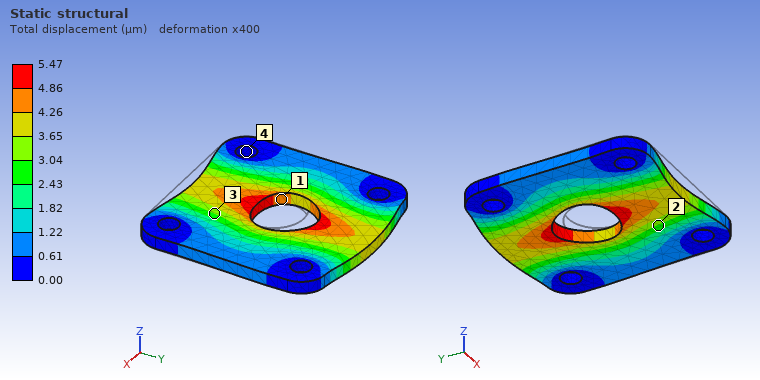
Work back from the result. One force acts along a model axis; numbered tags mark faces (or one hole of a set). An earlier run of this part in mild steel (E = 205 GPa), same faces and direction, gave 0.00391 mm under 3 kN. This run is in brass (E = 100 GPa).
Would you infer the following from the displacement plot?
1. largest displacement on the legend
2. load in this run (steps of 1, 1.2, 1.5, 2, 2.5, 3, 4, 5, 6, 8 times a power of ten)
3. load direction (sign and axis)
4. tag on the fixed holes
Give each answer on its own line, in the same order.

5.47 µm
2 kN
+Y
4
